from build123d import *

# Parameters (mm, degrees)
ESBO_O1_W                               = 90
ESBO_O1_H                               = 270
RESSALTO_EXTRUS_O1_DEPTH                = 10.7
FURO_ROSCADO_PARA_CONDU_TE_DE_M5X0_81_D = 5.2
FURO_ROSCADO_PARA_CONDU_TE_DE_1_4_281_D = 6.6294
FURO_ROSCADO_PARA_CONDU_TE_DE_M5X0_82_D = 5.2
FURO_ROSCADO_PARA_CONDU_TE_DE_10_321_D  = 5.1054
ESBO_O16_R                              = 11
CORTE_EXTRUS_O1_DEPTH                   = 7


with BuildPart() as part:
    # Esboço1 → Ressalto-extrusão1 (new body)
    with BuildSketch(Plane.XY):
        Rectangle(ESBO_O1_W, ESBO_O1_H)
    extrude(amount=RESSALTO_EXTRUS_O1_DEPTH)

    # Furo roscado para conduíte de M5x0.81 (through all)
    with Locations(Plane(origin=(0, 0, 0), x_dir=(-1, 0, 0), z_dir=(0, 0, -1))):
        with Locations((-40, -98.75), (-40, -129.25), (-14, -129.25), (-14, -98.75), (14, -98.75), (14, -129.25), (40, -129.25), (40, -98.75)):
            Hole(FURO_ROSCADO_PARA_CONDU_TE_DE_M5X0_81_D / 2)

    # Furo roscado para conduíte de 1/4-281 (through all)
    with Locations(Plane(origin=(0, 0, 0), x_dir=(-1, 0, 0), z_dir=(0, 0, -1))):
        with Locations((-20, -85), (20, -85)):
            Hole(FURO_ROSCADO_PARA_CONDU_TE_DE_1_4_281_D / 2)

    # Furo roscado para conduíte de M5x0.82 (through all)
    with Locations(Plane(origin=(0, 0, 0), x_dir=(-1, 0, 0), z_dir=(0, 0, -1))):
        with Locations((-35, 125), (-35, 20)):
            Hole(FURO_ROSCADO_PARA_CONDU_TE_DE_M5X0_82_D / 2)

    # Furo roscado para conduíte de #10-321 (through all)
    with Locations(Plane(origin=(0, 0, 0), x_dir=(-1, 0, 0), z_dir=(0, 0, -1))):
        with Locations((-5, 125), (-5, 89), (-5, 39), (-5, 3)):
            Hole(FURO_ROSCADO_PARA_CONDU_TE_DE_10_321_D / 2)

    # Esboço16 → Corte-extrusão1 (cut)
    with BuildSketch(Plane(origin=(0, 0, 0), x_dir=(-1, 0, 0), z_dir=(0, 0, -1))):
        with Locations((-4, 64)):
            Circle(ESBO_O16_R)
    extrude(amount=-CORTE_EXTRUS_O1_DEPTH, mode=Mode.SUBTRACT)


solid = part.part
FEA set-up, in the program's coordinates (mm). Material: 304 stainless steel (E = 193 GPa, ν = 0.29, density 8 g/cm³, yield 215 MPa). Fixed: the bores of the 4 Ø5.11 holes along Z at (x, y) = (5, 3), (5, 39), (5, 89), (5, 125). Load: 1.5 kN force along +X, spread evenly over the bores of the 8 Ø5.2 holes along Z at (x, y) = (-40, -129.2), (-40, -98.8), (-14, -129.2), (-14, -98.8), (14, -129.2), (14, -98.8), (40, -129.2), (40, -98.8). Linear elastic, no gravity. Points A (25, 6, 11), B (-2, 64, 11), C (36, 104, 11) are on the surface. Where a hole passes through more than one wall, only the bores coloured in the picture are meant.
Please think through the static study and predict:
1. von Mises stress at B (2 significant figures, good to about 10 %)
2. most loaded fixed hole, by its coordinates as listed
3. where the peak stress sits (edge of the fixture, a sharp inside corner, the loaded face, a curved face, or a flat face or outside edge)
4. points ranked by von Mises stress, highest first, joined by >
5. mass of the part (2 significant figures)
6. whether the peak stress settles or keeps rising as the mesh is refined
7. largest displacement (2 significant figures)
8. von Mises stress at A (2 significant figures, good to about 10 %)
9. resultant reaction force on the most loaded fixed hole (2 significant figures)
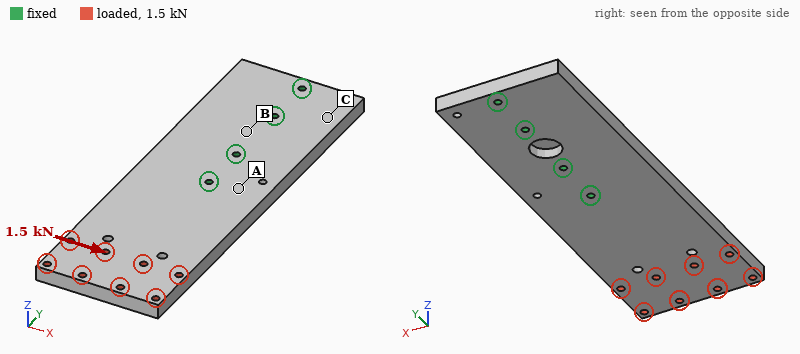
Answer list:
5.7 MPa
(5, 3)
edge of the fixture
A > B > C
2.0 kg
keeps rising
24 µm
8.2 MPa
3.6 kN
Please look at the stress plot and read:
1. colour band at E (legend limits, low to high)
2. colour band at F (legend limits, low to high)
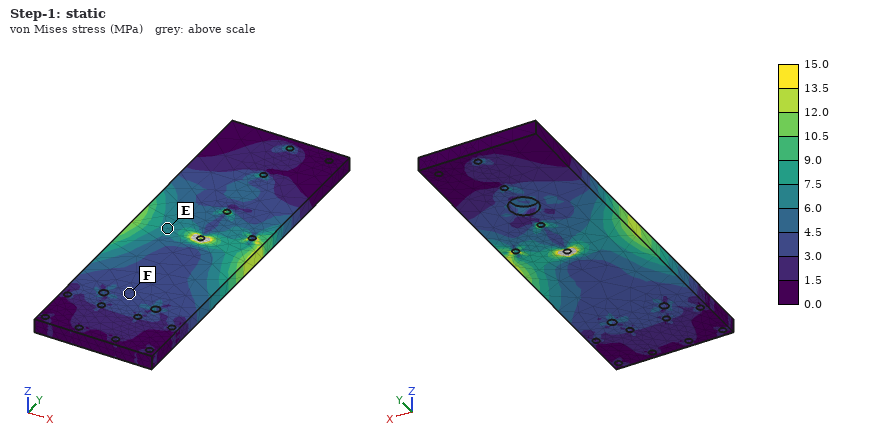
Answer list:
6.0 to 7.5 MPa
3.0 to 4.5 MPa
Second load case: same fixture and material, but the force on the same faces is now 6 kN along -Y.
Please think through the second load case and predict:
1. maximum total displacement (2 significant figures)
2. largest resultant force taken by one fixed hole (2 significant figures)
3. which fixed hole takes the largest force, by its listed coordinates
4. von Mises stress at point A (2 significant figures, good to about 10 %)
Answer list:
6.3 µm
3.5 kN
(5, 3)
4.3 MPa
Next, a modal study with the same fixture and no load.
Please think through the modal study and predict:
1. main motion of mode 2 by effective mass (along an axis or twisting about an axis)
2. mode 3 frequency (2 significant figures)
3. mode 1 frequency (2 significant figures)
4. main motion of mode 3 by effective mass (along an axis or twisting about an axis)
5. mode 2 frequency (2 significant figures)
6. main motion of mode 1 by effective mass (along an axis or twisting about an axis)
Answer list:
twisting about Y
2000 Hz
410 Hz
along X
1100 Hz
along Z
